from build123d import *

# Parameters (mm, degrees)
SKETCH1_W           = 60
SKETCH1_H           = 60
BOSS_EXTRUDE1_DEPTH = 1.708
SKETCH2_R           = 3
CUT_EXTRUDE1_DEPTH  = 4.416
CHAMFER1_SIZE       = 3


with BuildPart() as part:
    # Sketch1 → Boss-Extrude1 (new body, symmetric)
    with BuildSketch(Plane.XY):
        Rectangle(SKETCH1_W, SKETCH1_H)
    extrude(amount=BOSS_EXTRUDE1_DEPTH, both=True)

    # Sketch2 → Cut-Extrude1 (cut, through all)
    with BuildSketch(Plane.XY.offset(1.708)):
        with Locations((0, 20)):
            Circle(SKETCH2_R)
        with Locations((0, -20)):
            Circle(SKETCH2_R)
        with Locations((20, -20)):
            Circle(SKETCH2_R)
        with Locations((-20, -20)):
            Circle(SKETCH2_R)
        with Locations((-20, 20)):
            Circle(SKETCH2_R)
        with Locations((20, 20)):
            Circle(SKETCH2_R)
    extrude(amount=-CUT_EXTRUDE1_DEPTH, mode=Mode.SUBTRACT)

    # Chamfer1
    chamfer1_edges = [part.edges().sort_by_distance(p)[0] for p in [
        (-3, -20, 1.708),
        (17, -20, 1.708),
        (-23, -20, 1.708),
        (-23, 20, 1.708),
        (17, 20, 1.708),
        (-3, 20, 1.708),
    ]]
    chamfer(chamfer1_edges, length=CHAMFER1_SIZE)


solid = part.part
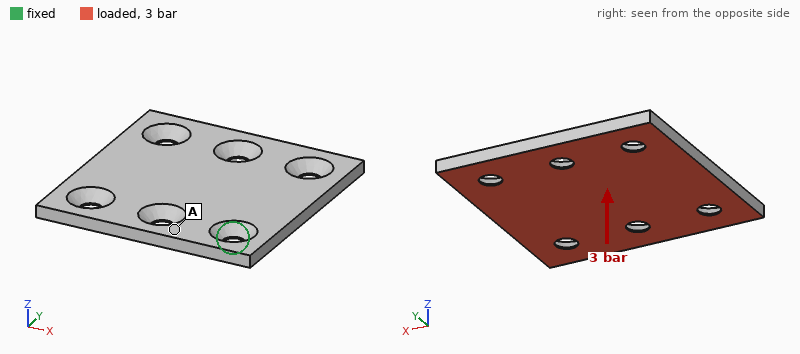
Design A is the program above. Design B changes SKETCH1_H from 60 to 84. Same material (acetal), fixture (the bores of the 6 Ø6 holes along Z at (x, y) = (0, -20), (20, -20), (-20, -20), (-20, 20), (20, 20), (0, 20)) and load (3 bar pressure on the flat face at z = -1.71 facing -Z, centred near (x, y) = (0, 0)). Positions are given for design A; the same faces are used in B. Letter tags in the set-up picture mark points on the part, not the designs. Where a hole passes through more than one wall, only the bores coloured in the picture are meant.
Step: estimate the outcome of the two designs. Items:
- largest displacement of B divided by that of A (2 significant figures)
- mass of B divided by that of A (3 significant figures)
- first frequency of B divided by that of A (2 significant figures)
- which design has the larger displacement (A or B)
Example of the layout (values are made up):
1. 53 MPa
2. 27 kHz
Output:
1. 3.6
2. 1.45
3. 0.48
4. B
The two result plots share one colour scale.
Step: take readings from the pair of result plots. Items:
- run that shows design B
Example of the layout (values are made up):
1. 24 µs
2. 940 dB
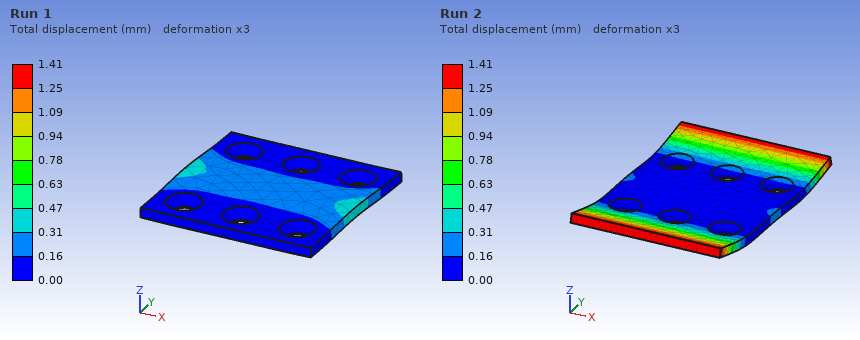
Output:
1. Run 2
